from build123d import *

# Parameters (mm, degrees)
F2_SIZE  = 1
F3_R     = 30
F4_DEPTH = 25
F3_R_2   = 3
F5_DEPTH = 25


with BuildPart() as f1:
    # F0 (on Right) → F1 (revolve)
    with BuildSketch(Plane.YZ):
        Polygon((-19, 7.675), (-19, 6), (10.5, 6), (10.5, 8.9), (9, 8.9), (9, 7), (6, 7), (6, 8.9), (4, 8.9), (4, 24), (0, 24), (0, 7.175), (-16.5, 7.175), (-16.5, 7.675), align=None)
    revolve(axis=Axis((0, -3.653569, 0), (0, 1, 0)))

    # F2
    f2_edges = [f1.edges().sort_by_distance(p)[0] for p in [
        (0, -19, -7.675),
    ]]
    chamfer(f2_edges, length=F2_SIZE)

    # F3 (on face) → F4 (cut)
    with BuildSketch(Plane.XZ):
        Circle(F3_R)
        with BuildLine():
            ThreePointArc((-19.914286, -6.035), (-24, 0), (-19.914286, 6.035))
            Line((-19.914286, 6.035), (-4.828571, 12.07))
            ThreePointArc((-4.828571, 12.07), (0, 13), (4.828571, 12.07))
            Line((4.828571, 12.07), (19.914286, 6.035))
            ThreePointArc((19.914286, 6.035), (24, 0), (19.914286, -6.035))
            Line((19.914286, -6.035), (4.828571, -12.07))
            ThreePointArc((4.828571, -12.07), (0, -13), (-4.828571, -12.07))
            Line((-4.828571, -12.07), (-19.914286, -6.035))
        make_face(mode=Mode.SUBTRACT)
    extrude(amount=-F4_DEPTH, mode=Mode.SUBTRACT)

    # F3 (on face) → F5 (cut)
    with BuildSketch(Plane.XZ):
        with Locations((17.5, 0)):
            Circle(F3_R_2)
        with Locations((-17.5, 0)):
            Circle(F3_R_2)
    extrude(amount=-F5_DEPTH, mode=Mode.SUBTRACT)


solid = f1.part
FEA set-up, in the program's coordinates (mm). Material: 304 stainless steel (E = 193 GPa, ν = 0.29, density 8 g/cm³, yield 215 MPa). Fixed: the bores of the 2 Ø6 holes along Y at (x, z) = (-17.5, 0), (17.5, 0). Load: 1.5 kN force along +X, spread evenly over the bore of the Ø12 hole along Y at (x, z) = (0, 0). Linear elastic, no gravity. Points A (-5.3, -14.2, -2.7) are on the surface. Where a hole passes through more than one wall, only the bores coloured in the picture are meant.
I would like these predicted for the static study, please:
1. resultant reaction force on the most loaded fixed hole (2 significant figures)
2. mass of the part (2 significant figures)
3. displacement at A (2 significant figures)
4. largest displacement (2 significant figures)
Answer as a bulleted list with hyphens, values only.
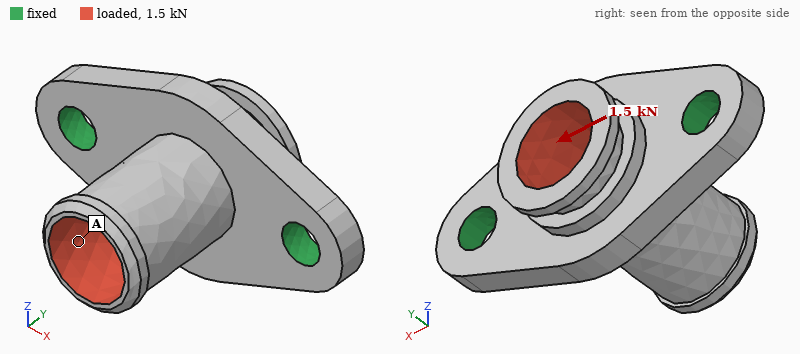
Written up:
- 850 N
- 35 g
- 15 µm
- 18 µm
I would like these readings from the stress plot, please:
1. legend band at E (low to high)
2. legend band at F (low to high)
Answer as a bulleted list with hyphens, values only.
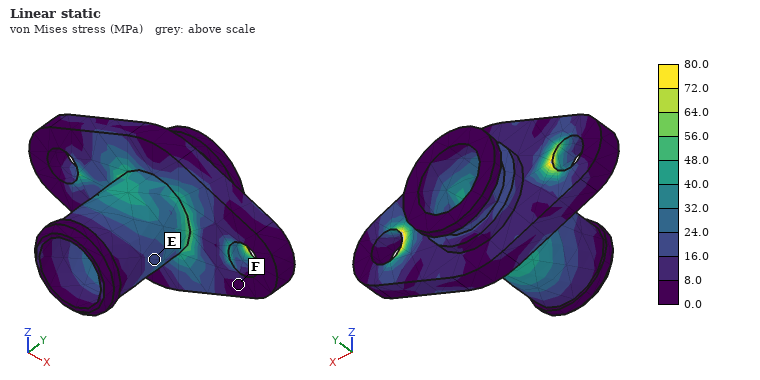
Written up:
- 16.0 to 24.0 MPa
- 0.0 to 8.0 MPa
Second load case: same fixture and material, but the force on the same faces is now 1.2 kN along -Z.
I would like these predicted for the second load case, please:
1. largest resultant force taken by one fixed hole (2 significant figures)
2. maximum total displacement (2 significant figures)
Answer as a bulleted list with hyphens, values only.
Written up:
- 600 N
- 36 µm
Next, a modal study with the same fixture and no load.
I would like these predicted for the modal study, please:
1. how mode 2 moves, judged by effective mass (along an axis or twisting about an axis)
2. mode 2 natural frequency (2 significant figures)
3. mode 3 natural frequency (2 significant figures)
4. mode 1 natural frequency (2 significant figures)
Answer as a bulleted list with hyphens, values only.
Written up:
- along Y
- 14 kHz
- 14 kHz
- 7800 Hz
